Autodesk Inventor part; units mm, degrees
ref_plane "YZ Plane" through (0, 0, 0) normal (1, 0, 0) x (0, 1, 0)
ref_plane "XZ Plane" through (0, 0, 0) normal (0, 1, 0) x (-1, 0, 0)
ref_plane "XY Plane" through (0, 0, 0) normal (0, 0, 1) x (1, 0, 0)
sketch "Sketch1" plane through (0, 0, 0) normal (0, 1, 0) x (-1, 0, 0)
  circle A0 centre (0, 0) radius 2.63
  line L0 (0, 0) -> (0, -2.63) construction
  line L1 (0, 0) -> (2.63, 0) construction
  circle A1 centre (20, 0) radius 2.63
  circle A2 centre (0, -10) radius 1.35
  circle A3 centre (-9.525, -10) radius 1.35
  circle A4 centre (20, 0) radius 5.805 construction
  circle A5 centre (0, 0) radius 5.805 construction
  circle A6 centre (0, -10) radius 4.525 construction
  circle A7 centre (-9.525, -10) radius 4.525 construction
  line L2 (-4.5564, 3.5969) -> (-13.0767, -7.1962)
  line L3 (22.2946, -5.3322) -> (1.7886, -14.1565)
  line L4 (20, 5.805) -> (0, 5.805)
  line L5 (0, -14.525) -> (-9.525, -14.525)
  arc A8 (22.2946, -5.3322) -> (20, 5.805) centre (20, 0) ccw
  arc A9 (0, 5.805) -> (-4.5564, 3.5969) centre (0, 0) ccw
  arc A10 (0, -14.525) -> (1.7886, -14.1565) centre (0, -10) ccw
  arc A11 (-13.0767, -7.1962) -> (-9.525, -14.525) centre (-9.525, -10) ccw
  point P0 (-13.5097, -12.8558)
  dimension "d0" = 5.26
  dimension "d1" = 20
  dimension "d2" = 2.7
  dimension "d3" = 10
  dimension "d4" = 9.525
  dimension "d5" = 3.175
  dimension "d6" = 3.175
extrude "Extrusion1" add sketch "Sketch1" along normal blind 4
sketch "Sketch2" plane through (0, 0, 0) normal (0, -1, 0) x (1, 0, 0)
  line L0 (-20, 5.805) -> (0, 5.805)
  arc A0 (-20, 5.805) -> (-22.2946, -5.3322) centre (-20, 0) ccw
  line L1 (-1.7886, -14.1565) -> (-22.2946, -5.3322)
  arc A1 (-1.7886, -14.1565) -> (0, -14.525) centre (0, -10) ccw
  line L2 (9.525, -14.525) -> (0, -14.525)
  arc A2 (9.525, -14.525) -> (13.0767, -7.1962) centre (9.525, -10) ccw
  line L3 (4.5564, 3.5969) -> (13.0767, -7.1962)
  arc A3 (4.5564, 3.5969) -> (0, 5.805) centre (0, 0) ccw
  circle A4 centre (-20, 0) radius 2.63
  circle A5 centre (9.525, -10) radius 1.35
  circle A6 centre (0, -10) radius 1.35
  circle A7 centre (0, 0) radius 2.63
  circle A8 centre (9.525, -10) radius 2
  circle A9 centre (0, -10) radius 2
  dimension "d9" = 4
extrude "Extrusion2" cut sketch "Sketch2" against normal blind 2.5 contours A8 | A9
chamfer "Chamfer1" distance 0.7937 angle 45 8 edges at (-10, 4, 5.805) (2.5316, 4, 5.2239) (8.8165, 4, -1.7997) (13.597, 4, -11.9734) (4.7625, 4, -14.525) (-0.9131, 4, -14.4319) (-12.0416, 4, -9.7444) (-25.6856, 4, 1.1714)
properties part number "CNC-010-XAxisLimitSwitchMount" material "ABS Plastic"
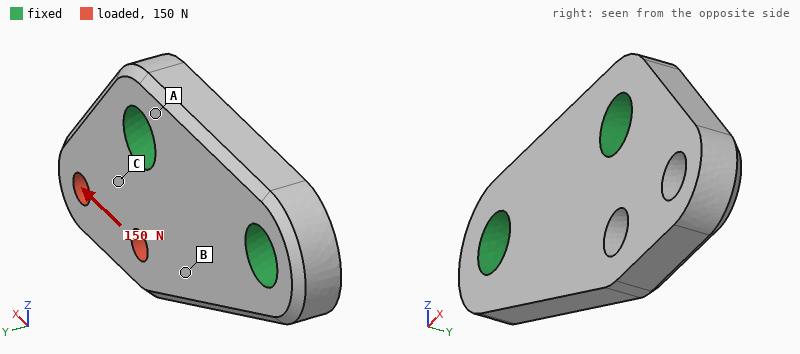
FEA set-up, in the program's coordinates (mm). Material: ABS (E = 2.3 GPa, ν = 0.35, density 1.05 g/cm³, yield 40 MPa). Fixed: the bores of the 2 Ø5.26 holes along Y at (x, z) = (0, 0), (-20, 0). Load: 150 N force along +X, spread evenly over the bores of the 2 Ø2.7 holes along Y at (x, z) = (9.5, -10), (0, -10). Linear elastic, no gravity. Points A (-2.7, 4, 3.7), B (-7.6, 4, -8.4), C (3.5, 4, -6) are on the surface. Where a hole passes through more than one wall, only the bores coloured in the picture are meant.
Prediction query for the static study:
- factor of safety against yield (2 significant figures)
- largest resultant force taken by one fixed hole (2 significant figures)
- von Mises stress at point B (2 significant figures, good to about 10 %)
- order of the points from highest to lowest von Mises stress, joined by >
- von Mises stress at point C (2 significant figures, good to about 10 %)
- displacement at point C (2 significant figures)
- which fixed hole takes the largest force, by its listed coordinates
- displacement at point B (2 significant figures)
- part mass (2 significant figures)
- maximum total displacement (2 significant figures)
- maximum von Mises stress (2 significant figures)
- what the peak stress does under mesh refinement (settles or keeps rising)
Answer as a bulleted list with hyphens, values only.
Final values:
- 2.2
- 110 N
- 4.4 MPa
- C > B > A
- 6.6 MPa
- 0.027 mm
- (0, 0)
- 0.018 mm
- 2.1 g
- 0.11 mm
- 18 MPa
- settles
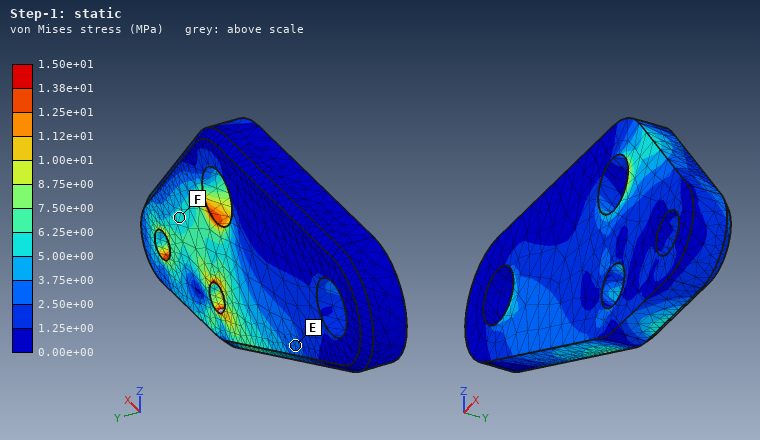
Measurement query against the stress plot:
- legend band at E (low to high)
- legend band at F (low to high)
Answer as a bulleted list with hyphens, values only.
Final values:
- 2.50e+00 to 3.75e+00 MPa
- 5.00e+00 to 6.25e+00 MPa
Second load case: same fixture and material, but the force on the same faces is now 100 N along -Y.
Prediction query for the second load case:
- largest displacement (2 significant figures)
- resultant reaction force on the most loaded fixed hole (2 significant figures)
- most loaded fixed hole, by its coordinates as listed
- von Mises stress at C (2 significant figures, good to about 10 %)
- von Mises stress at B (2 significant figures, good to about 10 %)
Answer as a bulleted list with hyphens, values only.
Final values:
- 0.38 mm
- 110 N
- (0, 0)
- 11 MPa
- 6.1 MPa
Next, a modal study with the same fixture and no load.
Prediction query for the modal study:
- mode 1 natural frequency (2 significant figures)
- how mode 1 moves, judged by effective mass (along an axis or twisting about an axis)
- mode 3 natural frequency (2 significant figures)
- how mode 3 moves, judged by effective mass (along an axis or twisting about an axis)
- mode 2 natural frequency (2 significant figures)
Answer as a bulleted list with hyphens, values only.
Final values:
- 4400 Hz
- along Y
- 10 kHz
- along X
- 7300 Hz
